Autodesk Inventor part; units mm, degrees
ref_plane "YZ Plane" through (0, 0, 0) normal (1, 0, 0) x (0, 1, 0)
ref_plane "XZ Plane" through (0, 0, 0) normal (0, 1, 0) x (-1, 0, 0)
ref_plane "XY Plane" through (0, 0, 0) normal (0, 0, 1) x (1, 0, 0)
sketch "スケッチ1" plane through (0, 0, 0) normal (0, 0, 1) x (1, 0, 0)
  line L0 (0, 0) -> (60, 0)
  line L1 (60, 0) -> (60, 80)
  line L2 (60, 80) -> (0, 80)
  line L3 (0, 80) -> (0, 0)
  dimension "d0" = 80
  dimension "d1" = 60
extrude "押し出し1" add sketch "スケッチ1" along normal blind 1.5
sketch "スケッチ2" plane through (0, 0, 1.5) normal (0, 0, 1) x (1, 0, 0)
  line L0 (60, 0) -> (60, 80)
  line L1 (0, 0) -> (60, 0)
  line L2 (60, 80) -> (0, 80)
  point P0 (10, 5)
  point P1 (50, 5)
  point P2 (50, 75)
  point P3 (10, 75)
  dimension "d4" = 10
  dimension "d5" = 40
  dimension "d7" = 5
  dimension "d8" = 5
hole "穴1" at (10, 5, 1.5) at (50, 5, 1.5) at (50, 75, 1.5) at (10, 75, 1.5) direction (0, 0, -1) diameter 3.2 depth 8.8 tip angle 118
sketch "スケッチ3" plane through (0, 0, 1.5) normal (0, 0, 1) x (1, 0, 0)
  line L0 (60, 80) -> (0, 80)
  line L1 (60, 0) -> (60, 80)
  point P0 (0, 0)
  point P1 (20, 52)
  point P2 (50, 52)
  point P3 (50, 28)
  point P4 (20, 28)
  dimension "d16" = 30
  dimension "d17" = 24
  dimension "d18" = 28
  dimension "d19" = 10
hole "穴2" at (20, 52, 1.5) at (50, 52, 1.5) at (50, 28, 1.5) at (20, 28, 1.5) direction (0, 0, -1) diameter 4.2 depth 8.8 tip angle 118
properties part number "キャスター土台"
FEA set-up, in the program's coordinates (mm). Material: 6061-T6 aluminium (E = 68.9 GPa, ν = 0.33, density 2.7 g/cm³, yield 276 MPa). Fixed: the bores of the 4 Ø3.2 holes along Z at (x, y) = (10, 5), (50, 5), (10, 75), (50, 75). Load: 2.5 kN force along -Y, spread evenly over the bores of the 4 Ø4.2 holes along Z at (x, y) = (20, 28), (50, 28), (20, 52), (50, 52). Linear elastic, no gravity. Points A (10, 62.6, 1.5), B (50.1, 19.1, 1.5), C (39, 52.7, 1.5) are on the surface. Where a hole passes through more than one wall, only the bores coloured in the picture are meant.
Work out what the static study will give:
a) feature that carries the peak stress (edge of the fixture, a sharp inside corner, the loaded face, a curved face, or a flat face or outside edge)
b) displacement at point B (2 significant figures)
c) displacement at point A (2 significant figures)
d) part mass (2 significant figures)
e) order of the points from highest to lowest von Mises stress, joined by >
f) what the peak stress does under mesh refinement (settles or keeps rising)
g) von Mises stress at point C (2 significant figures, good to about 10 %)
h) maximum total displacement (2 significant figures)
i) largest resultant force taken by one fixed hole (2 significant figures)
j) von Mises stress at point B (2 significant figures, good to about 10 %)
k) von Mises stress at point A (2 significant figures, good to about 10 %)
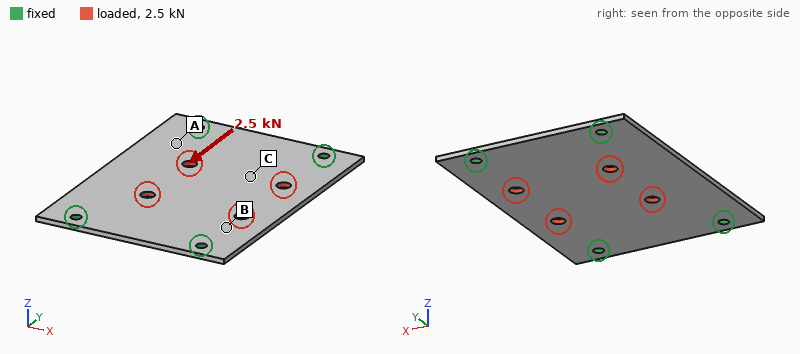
edge of the fixture
7.0 µm
4.7 µm
19 g
B > A > C
keeps rising
6.0 MPa
12 µm
700 N
28 MPa
19 MPa
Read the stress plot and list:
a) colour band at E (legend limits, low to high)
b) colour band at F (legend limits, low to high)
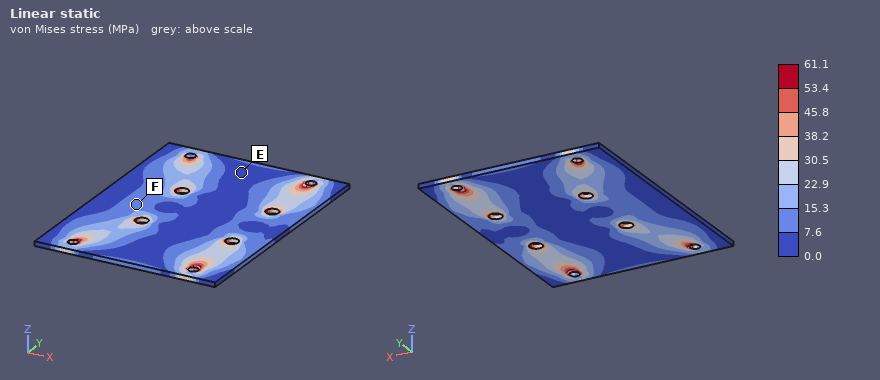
0.0 to 7.6 MPa
7.6 to 15.3 MPa
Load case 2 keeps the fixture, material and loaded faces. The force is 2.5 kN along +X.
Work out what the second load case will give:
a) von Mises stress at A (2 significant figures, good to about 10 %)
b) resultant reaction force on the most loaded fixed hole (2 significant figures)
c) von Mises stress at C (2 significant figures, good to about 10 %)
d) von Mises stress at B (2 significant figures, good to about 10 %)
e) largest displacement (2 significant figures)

20 MPa
710 N
23 MPa
22 MPa
24 µm
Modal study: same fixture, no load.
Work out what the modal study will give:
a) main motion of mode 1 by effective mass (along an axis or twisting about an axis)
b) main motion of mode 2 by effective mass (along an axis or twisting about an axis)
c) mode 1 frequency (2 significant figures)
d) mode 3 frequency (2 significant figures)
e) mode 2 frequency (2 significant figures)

along Z
twisting about Y
1500 Hz
3300 Hz
2000 Hz
